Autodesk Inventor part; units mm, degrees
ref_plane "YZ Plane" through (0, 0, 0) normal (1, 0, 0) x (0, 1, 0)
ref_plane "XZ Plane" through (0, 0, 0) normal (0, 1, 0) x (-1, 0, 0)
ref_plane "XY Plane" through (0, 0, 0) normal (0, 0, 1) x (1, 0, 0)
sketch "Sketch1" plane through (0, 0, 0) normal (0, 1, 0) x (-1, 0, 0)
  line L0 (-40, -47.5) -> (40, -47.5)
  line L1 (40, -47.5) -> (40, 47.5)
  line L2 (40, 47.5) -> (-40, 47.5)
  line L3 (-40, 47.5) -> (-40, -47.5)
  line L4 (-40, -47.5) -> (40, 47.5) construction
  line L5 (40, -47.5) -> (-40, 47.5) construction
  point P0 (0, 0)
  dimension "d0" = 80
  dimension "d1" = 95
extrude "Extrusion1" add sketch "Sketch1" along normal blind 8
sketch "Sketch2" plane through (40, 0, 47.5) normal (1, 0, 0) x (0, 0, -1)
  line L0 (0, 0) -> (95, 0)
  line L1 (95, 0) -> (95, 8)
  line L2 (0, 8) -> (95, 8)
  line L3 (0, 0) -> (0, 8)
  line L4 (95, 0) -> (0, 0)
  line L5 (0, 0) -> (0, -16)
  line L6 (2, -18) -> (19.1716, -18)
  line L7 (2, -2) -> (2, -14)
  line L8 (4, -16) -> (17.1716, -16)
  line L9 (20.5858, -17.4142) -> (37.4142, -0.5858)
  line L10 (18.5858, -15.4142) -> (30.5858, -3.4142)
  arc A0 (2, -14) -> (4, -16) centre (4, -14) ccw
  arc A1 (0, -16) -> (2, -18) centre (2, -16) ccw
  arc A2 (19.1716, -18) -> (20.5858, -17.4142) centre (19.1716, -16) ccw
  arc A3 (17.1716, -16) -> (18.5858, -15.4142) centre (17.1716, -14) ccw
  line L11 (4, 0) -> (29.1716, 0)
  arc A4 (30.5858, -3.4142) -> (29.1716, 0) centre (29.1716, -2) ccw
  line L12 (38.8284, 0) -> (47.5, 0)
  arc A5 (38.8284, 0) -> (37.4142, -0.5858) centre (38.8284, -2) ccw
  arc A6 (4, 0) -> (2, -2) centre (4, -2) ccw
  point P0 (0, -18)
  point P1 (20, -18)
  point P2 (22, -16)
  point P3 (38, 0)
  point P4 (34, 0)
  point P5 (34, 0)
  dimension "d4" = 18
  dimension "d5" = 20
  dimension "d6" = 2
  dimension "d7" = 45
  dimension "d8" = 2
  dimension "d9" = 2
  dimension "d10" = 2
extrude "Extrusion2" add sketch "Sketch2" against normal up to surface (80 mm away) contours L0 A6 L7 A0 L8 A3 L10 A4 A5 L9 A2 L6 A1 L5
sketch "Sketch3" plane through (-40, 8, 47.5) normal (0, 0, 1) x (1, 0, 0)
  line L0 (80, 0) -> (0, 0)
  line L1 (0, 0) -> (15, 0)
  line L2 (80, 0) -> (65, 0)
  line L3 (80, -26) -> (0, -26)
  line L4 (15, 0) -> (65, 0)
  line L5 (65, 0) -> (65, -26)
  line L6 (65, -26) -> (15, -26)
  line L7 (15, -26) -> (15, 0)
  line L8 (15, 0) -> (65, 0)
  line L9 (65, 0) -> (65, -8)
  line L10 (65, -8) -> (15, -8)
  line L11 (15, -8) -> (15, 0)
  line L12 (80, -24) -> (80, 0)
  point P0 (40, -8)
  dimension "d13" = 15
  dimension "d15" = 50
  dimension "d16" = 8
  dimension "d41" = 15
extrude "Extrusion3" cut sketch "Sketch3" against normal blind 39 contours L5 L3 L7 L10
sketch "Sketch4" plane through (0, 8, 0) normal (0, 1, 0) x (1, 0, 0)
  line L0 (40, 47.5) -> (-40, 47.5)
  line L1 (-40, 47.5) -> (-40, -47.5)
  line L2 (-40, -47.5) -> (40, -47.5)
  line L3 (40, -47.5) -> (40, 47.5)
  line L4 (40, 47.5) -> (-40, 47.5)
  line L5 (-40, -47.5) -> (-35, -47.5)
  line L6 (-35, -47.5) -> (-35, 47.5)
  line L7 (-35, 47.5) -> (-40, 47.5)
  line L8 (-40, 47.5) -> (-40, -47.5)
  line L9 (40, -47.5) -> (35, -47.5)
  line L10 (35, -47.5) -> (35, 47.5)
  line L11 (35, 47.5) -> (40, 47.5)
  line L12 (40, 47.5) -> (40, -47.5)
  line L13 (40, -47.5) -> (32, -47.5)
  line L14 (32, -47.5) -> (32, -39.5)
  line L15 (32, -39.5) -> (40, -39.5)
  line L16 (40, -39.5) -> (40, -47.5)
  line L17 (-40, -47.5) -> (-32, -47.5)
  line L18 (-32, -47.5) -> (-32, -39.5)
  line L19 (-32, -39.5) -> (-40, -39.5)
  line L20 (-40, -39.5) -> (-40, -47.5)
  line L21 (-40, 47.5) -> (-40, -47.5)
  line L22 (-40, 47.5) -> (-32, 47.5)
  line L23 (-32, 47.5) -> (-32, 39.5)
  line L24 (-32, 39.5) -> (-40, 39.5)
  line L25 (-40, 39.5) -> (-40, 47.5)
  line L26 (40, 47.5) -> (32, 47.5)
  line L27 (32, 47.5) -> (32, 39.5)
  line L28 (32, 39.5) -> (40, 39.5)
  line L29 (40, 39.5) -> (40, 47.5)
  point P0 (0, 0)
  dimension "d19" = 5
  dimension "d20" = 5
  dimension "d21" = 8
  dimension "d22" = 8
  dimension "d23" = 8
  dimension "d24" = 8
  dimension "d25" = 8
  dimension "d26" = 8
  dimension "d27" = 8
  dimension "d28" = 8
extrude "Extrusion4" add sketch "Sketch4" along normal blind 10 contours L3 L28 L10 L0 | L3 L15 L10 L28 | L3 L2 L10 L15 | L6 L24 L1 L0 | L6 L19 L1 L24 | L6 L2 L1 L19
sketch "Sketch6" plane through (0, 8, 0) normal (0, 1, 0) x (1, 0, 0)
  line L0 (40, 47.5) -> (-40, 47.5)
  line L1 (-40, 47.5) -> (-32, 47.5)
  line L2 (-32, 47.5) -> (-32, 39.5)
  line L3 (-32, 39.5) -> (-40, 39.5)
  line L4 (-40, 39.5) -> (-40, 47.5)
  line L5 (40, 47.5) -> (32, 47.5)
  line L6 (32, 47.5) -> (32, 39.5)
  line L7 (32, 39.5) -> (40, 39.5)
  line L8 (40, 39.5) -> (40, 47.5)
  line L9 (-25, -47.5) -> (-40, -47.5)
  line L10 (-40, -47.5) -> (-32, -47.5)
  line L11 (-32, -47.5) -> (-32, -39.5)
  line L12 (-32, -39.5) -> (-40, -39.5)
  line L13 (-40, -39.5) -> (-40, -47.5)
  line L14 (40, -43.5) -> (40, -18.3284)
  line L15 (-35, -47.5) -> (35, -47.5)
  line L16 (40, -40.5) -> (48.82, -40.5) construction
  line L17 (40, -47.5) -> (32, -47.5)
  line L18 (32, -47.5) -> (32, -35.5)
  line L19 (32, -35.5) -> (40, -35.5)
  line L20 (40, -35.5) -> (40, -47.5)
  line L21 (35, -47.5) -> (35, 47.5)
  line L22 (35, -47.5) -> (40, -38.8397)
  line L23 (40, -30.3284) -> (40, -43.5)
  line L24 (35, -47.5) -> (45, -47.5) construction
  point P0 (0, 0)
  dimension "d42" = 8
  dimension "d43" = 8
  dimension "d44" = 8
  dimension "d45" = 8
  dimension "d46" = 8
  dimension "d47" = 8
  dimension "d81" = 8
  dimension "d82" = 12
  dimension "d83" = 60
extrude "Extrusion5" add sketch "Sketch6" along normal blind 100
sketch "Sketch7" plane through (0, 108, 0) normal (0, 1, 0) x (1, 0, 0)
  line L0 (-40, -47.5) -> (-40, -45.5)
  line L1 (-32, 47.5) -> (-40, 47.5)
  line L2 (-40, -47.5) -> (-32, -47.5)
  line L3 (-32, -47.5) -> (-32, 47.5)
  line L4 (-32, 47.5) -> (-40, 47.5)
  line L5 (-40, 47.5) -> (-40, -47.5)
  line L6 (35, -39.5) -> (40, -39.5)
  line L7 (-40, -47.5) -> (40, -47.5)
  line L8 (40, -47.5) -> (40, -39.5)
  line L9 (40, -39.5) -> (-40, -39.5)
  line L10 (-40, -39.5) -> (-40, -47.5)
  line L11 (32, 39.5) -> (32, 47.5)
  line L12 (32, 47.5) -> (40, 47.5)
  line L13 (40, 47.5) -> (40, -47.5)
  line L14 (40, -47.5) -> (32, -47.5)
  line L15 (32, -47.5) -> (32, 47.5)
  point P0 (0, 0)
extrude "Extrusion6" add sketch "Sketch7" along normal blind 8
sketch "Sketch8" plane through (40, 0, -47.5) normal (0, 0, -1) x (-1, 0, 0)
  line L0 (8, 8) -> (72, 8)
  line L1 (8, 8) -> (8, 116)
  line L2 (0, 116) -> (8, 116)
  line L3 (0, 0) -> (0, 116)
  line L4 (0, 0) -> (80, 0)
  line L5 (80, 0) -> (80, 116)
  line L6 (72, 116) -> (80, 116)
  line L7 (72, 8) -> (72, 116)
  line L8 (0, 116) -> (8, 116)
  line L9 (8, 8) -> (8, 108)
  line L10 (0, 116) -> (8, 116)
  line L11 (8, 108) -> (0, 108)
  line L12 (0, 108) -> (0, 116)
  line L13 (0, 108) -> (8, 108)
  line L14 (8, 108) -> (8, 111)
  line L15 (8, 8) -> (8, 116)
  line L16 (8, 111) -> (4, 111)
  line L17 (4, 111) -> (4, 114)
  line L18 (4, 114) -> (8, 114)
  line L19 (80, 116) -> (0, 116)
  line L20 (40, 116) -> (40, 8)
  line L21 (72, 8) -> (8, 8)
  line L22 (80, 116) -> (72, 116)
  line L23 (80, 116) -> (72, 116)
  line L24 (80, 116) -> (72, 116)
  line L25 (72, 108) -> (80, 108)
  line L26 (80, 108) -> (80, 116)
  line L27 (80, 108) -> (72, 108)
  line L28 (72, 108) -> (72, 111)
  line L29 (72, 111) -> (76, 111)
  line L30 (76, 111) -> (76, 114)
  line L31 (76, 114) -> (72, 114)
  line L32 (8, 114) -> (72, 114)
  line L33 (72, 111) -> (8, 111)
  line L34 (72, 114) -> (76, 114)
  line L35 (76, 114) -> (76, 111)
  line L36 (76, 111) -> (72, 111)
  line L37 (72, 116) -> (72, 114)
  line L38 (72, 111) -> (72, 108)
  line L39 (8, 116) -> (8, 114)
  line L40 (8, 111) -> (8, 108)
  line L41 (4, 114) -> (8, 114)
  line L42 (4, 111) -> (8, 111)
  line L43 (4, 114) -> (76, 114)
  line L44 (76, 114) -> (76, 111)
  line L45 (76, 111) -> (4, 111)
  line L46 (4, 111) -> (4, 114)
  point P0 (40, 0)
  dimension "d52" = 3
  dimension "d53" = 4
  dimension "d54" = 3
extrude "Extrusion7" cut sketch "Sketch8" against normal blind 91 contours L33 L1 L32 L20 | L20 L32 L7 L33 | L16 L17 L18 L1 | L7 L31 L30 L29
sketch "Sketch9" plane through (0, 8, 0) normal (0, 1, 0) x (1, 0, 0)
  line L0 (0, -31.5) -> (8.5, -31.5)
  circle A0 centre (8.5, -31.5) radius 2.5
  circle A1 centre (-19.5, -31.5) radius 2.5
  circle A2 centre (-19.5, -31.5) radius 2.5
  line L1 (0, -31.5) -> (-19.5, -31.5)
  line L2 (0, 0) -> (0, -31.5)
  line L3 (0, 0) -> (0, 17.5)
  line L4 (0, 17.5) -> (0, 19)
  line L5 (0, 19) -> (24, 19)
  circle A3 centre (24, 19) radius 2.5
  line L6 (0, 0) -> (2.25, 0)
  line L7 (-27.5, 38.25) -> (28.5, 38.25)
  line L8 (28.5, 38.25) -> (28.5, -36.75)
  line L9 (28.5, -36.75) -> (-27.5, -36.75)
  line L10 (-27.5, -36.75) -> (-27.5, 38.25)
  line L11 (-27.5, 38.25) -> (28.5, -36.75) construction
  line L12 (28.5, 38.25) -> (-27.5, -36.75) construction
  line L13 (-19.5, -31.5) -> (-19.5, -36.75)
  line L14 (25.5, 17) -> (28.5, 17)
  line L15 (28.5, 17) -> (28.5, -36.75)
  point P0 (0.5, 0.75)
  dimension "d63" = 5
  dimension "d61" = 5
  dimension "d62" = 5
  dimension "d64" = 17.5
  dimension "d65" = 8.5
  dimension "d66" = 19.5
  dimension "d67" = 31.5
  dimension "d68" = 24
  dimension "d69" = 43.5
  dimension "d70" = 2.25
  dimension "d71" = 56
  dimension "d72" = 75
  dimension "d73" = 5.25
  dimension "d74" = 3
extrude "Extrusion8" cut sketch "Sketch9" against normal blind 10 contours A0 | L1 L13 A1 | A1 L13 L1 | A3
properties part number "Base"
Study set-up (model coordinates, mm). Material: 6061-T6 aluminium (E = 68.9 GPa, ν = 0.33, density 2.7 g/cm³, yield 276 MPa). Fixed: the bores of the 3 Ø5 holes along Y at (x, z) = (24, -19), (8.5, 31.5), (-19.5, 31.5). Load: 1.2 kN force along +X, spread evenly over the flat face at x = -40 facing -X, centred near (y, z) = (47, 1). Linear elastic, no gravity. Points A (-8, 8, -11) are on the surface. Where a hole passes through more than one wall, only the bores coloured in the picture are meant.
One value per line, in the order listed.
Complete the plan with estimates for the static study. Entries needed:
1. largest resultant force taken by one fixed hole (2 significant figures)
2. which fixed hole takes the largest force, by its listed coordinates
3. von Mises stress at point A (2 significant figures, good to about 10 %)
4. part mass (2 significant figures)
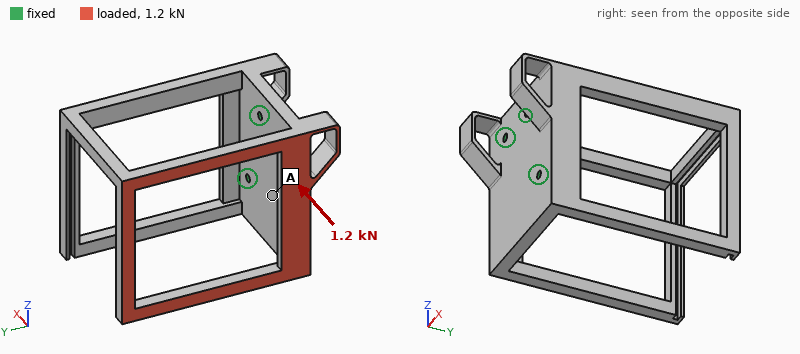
980 N
(-19.5, 31.5)
14 MPa
310 g
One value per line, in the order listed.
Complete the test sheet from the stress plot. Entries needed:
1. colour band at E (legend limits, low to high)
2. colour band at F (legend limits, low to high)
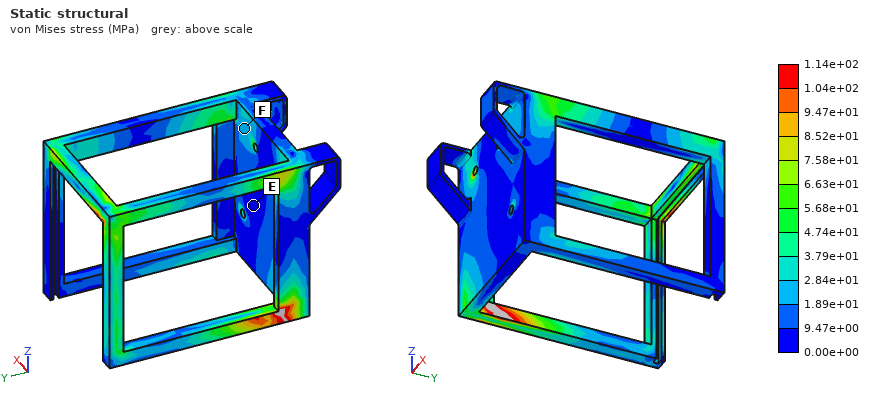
0.00e+00 to 9.47e+00 MPa
1.89e+01 to 2.84e+01 MPa
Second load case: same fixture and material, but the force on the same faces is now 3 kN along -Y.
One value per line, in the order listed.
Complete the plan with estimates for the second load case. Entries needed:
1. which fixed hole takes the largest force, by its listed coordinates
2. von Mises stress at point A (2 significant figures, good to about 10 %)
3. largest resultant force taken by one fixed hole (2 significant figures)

(-19.5, 31.5)
45 MPa
3.4 kN
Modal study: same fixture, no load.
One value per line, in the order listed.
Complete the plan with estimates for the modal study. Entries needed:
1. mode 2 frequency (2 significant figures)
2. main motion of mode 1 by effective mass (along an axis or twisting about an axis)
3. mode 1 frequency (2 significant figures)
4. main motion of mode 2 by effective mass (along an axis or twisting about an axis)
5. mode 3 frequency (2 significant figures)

580 Hz
along X
440 Hz
along Z
650 Hz
